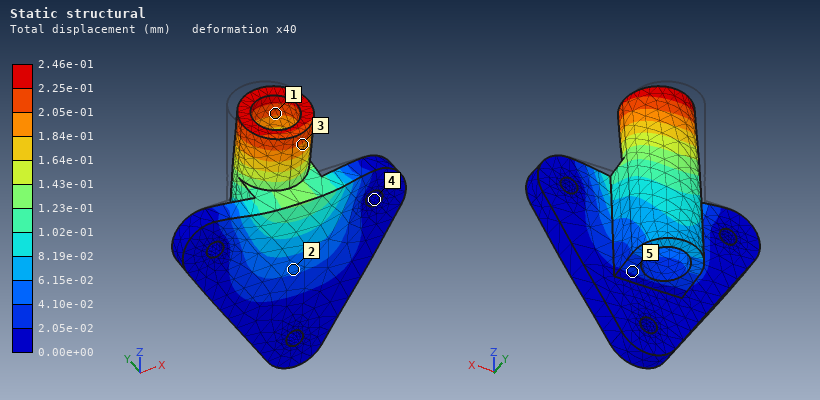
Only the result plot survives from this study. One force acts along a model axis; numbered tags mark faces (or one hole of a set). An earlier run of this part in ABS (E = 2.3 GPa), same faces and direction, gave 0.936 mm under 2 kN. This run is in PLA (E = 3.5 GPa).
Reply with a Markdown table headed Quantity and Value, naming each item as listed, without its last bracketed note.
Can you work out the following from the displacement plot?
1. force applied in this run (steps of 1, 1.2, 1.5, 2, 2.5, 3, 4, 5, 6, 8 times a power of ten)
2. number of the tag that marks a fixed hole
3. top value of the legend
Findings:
| Quantity | Value |
|---|---|
| force applied in this run | 800 N |
| number of the tag that marks a fixed hole | 4 |
| top value of the legend | 2.46e-01 mm |
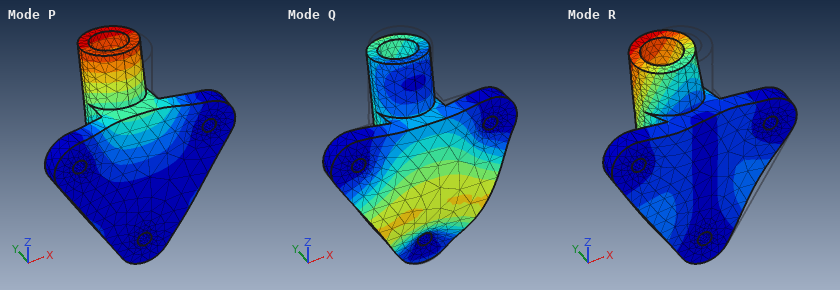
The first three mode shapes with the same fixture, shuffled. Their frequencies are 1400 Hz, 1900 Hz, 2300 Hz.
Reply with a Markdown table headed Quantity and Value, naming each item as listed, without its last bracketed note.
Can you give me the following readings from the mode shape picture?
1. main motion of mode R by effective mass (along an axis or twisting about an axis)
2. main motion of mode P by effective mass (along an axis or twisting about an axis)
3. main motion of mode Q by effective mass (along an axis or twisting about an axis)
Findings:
| Quantity | Value |
|---|---|
| main motion of mode R by effective mass | along X |
| main motion of mode P by effective mass | along Y |
| main motion of mode Q by effective mass | along Y |
